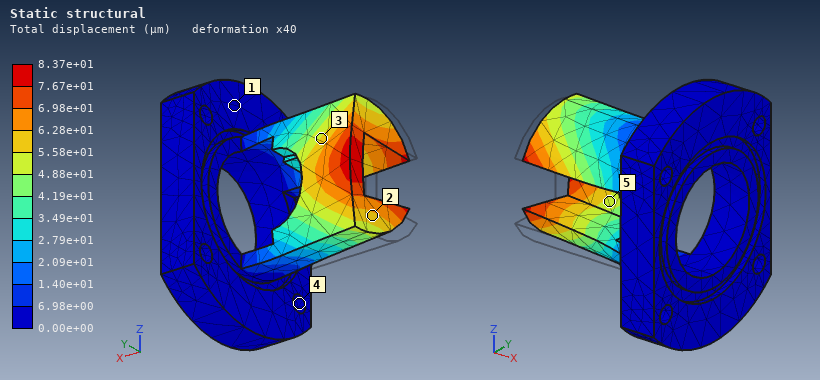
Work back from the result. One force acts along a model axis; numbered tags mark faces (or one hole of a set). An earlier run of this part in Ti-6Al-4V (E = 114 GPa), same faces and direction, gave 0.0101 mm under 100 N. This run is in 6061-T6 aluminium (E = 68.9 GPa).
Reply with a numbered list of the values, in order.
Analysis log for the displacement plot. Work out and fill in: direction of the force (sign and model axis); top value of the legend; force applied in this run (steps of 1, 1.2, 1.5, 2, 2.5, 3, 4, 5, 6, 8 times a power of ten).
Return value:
1. +Y
2. 8.37e+01 µm
3. 500 N
